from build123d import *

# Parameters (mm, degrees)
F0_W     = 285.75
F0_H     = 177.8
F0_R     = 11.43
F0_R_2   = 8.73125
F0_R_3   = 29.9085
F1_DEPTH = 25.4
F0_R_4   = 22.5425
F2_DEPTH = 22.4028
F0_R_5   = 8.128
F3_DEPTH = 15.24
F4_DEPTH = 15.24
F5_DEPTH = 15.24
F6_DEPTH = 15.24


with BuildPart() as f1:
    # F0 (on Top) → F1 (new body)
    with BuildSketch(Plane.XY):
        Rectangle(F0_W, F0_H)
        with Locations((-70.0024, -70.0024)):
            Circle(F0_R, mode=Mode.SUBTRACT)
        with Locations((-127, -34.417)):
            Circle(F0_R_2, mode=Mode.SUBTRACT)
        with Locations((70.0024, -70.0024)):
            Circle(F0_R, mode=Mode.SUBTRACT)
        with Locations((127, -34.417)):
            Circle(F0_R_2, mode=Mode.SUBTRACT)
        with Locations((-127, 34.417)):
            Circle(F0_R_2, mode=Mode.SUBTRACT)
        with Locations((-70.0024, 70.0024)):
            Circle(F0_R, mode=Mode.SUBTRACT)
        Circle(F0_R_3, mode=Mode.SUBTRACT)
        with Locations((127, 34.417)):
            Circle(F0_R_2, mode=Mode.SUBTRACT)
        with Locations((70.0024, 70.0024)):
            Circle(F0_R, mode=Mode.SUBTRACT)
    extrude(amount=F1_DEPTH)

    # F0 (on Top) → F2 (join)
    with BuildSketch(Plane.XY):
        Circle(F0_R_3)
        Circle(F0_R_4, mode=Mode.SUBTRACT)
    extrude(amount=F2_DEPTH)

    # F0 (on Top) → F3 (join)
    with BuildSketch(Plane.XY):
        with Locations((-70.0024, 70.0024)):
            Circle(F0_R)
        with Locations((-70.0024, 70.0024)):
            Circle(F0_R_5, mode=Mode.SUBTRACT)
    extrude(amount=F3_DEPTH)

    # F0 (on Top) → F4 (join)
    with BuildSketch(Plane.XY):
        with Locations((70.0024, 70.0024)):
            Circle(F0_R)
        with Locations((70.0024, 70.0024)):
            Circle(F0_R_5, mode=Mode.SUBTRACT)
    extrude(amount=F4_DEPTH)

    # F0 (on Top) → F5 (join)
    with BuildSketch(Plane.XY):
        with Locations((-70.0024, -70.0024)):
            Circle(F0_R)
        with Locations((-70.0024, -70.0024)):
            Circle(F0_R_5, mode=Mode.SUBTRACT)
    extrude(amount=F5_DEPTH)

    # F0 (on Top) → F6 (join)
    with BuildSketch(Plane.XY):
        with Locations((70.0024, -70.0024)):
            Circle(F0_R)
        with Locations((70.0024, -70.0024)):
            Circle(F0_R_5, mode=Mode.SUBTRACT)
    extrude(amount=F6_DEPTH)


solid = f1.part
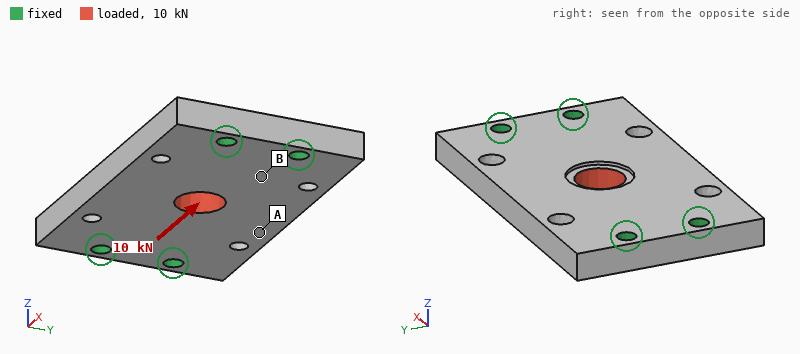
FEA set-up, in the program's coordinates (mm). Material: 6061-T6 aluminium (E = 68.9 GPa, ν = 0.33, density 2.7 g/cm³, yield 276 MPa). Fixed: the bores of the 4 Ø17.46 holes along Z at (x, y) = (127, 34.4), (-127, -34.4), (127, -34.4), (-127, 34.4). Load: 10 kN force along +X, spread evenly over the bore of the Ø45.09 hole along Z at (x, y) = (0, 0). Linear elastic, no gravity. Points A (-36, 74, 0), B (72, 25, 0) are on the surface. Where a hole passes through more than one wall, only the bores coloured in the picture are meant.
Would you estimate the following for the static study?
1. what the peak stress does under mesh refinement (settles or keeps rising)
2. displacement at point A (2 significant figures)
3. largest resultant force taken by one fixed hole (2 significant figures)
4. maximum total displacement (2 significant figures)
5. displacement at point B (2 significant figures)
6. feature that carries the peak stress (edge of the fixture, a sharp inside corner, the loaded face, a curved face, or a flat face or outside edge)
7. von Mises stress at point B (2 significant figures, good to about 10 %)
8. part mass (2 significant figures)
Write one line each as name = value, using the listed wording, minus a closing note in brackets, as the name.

what the peak stress does under mesh refinement = keeps rising
displacement at point A = 1.7 µm
largest resultant force taken by one fixed hole = 2.5 kN
maximum total displacement = 3.7 µm
displacement at point B = 1.5 µm
feature that carries the peak stress = a sharp inside corner
von Mises stress at point B = 2.0 MPa
part mass = 3.2 kg
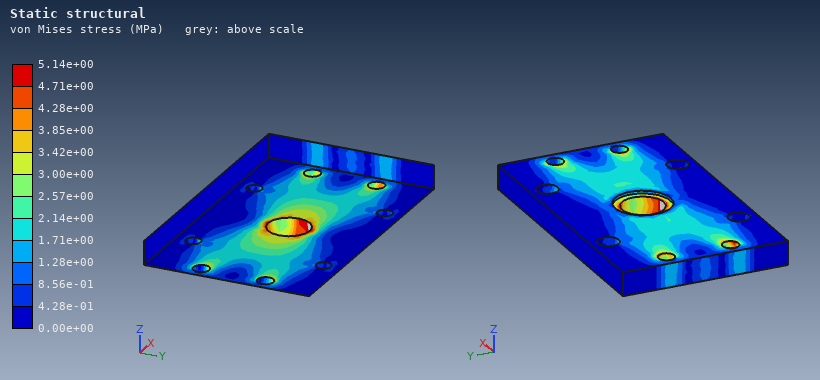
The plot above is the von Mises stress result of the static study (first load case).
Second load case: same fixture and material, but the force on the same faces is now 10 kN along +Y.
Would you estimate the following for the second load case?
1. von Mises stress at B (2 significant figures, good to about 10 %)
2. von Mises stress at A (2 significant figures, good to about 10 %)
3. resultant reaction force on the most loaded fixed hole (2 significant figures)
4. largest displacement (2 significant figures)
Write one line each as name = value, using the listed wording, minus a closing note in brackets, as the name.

von Mises stress at B = 3.1 MPa
von Mises stress at A = 2.0 MPa
resultant reaction force on the most loaded fixed hole = 3.2 kN
largest displacement = 9.5 µm
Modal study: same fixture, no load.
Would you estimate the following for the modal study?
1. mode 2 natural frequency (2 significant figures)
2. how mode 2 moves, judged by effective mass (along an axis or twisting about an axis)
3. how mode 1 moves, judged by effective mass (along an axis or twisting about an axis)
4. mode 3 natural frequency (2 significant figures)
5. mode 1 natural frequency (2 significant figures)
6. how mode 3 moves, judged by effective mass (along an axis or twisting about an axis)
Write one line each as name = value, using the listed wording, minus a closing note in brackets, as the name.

mode 2 natural frequency = 2100 Hz
how mode 2 moves, judged by effective mass = twisting about X
how mode 1 moves, judged by effective mass = along Z
mode 3 natural frequency = 4400 Hz
mode 1 natural frequency = 1800 Hz
how mode 3 moves, judged by effective mass = twisting about Y
